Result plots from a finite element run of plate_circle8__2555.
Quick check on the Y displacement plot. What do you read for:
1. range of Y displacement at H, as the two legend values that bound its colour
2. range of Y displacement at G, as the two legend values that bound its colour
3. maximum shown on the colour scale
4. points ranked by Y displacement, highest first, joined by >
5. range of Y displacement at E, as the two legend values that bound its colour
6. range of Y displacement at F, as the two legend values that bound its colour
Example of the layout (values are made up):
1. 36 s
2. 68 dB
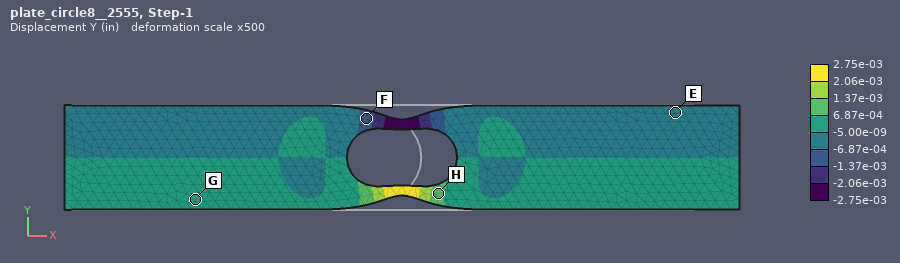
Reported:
1. 6.87e-04 to 1.37e-03 in
2. -5.00e-09 to 6.87e-04 in
3. 2.75e-03 in
4. H > G > E > F
5. -6.87e-04 to -5.00e-09 in
6. -1.37e-03 to -6.87e-04 in
